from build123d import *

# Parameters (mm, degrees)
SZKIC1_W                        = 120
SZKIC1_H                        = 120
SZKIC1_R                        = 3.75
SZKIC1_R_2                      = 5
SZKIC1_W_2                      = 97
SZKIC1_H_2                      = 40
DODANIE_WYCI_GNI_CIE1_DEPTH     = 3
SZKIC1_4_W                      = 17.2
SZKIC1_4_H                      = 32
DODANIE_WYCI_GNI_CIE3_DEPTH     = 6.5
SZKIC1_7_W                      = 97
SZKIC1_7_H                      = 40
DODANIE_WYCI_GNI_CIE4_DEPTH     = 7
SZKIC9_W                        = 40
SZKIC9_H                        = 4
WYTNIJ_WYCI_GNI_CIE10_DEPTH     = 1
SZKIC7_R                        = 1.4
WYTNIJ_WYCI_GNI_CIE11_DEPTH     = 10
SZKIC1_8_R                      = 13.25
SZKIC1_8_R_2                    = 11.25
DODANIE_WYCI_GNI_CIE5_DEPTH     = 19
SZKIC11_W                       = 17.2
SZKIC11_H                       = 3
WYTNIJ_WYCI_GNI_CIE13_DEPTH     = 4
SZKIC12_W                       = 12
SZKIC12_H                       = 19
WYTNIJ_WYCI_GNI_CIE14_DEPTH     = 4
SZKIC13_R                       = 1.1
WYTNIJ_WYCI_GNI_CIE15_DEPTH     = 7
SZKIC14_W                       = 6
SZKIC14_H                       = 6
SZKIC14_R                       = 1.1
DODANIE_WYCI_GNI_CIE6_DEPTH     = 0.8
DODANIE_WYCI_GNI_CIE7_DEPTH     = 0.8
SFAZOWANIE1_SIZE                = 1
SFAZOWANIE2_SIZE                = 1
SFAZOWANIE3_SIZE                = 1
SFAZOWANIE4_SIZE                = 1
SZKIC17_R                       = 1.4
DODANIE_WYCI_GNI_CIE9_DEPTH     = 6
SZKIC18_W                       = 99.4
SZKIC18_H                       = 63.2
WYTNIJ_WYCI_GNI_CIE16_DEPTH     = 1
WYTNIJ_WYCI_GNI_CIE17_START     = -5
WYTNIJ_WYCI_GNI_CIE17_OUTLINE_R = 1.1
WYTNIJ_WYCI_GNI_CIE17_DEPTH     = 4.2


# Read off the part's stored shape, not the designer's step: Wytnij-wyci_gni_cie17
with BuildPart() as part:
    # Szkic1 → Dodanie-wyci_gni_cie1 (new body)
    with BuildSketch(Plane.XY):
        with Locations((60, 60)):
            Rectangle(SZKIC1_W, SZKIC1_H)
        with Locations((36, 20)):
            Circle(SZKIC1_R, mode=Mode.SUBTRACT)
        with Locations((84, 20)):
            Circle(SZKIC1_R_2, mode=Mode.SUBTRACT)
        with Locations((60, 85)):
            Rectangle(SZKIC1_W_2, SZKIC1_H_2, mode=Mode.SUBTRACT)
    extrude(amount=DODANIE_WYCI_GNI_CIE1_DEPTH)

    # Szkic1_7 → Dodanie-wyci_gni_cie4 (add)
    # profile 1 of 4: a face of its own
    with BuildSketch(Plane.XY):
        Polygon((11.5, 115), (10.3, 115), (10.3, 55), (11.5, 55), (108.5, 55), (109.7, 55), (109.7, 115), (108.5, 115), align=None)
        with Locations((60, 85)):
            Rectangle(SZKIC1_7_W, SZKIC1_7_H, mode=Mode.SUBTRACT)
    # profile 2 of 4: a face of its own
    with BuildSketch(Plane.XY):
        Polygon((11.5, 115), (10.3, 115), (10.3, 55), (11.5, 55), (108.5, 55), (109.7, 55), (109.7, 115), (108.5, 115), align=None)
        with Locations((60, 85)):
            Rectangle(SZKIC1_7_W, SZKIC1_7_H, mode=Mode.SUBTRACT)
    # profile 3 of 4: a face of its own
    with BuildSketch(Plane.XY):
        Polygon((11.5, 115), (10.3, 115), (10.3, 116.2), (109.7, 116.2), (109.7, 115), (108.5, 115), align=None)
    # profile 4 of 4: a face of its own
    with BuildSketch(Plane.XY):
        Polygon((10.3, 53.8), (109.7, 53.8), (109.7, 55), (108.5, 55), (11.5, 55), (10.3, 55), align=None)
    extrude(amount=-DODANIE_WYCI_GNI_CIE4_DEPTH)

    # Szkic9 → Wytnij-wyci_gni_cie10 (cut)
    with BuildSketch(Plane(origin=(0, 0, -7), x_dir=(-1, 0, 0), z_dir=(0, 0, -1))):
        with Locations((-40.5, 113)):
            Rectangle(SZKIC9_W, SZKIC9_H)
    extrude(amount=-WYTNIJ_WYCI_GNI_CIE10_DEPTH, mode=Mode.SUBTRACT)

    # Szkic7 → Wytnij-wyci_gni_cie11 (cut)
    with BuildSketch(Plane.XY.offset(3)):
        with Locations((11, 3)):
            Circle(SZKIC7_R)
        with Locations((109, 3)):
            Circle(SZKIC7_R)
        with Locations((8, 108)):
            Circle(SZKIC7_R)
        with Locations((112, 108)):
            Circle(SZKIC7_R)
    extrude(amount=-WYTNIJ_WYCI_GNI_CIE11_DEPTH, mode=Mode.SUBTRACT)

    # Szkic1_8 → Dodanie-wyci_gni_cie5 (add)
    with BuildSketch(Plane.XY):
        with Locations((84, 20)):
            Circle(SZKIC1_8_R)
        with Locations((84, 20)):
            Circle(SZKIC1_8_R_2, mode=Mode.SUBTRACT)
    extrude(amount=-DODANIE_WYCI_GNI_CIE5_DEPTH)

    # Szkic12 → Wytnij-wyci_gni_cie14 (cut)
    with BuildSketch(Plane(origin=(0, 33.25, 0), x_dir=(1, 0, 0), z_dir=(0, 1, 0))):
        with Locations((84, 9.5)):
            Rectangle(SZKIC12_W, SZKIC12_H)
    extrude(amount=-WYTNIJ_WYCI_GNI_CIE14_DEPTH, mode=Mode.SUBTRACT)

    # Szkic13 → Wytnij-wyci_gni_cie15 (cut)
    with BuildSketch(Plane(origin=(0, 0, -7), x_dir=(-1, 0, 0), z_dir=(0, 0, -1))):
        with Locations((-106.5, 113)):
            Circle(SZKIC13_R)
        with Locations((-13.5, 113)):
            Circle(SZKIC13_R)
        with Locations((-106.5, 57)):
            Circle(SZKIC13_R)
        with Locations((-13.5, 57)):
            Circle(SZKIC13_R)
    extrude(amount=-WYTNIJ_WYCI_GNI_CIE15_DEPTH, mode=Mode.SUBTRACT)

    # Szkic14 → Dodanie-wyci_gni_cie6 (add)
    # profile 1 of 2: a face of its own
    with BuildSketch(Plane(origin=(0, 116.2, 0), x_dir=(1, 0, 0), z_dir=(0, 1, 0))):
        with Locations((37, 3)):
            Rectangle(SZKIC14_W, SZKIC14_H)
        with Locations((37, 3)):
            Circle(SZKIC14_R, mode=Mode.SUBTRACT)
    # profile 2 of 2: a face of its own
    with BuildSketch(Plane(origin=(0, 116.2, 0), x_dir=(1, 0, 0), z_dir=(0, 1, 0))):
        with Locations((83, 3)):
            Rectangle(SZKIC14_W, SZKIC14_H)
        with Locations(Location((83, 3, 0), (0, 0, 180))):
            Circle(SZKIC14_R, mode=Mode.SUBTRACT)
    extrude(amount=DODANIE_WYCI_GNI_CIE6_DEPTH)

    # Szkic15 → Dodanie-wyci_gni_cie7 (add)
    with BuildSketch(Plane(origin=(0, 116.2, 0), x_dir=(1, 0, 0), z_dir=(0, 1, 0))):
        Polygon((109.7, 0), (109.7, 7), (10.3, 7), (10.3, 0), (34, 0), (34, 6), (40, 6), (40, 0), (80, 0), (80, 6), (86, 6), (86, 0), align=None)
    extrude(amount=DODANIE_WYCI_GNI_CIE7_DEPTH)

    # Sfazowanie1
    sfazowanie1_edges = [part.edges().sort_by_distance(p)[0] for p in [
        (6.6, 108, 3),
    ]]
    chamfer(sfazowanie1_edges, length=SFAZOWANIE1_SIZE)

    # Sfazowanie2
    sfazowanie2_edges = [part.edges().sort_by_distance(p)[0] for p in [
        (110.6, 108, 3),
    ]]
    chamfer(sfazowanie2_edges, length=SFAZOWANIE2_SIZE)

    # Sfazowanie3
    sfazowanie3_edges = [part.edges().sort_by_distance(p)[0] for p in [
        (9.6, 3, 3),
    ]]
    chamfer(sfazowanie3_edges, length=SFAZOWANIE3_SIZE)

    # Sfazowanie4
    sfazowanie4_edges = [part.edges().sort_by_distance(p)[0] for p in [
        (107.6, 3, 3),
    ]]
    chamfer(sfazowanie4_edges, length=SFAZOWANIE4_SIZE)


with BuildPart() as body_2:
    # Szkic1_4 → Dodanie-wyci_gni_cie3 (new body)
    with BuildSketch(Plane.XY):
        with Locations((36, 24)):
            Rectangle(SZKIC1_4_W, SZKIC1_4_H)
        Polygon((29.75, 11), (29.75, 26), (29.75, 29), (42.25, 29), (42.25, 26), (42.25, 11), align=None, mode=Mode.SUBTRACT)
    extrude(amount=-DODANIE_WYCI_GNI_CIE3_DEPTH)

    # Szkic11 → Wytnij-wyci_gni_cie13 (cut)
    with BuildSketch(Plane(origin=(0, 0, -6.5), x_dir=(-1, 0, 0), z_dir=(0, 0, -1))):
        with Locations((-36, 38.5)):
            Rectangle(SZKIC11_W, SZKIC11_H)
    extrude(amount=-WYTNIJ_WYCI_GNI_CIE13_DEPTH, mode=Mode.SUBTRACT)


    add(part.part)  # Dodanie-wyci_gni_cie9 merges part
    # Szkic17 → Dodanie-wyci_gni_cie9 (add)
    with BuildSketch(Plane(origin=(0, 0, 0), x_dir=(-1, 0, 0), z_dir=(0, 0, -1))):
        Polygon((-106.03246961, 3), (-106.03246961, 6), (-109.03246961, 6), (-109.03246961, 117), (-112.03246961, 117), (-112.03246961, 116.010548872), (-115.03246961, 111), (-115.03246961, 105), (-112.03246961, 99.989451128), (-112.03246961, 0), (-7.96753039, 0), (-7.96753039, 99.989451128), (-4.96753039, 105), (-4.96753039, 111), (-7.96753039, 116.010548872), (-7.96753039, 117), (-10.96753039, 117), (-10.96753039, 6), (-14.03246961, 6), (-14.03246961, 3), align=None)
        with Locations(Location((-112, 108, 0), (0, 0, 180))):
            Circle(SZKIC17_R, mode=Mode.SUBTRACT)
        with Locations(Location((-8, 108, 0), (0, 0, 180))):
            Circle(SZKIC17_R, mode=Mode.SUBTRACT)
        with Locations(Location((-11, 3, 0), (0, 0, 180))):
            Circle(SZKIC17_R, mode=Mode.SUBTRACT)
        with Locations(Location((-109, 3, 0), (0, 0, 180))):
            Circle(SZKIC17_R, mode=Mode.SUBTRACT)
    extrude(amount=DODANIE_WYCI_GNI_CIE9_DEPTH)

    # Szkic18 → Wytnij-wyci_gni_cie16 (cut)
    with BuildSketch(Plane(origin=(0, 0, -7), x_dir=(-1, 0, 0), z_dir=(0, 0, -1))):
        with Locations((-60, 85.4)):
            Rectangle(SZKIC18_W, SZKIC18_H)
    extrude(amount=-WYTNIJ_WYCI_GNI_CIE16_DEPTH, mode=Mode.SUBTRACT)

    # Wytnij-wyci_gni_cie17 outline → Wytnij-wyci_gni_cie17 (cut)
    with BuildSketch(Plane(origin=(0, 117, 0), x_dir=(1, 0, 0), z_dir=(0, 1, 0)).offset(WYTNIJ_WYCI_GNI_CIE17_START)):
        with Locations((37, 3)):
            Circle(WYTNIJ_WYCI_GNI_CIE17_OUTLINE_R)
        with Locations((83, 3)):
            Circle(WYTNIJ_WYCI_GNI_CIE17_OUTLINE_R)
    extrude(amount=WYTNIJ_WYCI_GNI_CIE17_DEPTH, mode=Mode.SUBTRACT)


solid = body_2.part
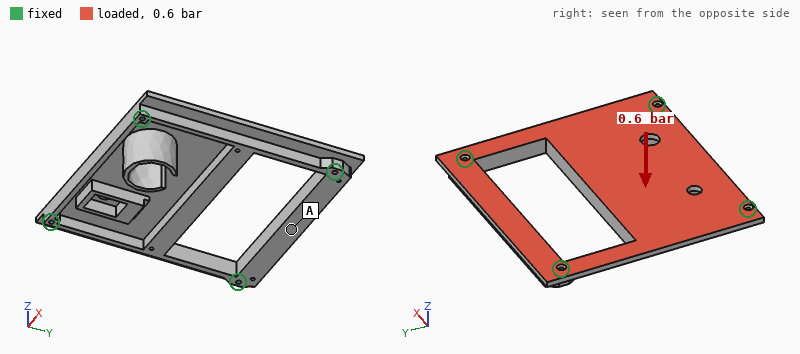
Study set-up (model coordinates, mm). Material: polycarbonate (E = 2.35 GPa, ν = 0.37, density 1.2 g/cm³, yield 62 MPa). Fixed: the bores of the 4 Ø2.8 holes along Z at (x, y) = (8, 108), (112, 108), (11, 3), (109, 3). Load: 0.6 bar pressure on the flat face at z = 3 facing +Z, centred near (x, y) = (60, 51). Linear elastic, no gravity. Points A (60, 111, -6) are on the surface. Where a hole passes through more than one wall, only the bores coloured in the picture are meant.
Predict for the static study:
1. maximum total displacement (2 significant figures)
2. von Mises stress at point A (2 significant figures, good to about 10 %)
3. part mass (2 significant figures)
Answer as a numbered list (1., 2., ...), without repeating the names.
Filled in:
1. 1.9 mm
2. 2.7 MPa
3. 67 g
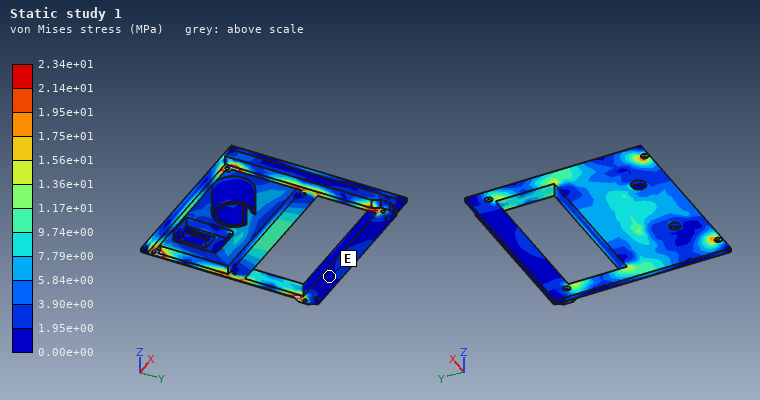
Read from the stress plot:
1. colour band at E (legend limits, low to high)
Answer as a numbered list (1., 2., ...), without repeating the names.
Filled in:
1. 0.00e+00 to 1.95e+00 MPa
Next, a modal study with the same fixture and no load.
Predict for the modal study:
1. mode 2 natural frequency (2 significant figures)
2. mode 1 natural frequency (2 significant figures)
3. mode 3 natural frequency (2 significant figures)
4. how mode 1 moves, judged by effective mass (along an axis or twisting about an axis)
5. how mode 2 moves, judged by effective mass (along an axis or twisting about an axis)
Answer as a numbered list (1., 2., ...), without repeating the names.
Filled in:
1. 760 Hz
2. 420 Hz
3. 890 Hz
4. along Z
5. twisting about Y
